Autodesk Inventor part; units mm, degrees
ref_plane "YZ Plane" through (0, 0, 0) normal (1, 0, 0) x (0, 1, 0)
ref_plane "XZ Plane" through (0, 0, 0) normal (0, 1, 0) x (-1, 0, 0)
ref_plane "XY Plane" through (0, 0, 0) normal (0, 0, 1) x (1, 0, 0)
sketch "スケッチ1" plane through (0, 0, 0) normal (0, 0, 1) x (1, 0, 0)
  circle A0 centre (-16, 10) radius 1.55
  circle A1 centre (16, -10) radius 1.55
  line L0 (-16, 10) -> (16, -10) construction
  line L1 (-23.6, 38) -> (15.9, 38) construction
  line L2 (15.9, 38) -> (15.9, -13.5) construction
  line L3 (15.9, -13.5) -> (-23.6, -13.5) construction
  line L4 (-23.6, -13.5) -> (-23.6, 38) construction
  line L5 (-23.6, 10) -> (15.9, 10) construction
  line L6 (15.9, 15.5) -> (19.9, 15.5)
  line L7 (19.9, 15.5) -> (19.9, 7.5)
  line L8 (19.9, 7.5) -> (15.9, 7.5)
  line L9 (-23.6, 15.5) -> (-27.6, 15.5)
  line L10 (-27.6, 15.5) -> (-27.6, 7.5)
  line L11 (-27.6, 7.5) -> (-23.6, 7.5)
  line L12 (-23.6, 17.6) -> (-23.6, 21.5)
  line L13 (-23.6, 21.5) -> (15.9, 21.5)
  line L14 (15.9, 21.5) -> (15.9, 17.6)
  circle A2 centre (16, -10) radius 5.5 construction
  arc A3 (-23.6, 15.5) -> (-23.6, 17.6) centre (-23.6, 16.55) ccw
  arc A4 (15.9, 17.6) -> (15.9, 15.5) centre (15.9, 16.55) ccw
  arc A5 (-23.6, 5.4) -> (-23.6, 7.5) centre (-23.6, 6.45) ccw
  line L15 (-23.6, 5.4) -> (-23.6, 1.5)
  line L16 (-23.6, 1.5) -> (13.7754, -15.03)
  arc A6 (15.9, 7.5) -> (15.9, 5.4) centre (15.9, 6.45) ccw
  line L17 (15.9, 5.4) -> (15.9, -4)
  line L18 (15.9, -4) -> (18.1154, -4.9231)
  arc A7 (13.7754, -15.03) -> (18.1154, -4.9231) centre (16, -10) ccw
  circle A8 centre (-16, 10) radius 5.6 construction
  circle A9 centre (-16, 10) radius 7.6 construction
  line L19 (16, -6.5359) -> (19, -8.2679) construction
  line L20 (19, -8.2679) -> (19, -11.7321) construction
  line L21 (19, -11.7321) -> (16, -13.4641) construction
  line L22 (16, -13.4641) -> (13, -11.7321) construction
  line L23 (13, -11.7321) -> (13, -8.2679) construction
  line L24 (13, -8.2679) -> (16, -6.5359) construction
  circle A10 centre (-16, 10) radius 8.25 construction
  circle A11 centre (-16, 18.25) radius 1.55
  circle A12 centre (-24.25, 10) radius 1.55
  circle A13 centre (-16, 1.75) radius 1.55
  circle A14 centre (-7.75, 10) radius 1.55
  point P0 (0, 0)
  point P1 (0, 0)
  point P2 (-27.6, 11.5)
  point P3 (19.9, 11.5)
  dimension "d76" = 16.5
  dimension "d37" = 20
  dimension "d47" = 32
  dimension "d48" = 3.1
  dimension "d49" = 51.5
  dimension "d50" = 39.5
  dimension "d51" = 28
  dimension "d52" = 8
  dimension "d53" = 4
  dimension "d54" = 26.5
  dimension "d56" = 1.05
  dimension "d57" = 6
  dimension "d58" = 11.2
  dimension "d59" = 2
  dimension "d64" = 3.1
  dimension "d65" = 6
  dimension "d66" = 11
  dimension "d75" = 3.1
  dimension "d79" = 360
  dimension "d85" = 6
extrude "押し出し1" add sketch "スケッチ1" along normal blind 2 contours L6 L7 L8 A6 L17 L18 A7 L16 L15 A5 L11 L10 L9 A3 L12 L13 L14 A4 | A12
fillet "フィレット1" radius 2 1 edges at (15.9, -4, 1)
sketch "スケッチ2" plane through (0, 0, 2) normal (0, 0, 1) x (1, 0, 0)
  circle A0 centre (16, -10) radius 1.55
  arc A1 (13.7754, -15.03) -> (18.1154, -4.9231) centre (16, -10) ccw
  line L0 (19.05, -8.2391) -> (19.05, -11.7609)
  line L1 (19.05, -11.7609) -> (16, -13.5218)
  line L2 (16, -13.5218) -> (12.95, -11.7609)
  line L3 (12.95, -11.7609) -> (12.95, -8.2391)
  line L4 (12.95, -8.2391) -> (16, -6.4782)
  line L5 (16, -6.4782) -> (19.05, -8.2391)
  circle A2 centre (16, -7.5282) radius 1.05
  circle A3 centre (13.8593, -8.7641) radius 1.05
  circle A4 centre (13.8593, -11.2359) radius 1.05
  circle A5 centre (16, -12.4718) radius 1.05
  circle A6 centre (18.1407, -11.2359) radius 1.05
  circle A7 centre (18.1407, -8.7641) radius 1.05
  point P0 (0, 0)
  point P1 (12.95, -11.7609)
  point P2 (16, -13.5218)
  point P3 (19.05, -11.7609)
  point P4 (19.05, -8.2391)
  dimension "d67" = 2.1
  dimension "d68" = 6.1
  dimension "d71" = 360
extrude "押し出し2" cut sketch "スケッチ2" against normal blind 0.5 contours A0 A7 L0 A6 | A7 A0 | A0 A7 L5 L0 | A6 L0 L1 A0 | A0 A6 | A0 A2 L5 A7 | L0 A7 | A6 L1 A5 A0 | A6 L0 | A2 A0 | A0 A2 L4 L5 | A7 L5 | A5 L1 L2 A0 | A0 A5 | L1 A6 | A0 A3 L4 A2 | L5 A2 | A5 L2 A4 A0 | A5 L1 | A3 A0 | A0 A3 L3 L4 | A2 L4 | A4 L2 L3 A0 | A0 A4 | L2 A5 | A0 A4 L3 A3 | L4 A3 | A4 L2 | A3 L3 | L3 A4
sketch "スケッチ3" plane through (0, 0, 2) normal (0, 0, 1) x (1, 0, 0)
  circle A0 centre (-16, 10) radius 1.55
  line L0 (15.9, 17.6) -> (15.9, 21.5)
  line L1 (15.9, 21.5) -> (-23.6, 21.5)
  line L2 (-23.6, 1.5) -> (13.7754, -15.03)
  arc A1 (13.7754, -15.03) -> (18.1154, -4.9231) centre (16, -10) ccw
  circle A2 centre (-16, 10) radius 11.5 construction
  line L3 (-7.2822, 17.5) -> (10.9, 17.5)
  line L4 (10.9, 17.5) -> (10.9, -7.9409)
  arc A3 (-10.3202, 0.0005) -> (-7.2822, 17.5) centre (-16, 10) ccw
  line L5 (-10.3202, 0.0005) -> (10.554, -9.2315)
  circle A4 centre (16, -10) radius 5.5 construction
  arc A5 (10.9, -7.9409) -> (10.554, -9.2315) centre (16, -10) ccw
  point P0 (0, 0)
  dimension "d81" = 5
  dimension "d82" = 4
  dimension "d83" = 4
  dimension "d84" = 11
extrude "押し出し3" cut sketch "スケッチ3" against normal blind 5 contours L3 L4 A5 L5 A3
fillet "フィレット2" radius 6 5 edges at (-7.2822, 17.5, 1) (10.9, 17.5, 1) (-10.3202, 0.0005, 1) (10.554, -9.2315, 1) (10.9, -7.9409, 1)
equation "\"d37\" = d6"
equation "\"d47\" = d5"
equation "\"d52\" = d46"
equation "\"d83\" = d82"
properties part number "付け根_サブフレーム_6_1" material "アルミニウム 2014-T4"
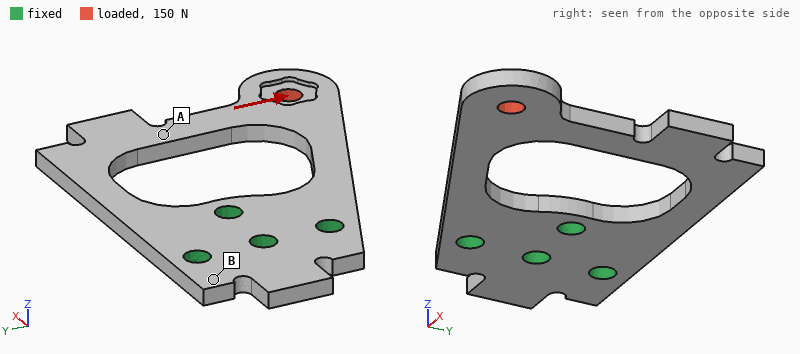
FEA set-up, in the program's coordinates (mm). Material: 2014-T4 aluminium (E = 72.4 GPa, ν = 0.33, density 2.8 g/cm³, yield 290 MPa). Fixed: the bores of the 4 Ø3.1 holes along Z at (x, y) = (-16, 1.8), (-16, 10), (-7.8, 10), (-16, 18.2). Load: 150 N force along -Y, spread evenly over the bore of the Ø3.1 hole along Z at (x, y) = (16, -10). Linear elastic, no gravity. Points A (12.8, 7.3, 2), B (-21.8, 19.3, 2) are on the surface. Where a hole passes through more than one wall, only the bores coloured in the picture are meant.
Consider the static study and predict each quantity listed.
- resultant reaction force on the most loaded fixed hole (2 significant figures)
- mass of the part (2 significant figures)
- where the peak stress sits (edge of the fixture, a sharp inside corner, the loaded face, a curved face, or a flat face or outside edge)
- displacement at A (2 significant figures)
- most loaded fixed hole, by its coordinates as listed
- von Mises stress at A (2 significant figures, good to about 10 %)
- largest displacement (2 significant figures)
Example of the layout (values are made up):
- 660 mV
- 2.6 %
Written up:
- 280 N
- 4.8 g
- a curved face
- 65 µm
- (-7.8, 10)
- 20 MPa
- 98 µm
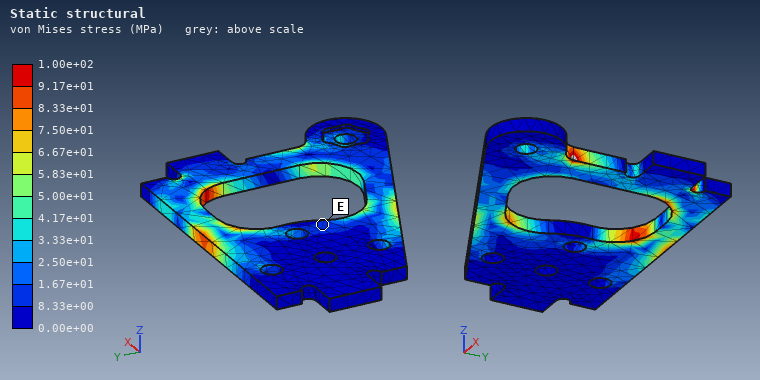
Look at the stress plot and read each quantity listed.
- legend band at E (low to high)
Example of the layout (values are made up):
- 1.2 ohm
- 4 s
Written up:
- 8.33e+00 to 1.67e+01 MPa
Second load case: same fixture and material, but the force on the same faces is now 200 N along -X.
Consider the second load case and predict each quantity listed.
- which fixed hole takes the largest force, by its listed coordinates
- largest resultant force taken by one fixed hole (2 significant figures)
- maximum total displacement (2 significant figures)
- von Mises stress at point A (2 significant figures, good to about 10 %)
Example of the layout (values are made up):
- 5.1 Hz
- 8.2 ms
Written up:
- (-16, 1.8)
- 270 N
- 84 µm
- 13 MPa
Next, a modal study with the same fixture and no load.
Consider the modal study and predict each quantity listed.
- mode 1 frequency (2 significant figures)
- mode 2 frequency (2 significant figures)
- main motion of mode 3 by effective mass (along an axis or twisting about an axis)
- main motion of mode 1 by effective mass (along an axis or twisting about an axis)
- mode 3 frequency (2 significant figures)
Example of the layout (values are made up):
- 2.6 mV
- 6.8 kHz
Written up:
- 1100 Hz
- 2400 Hz
- along Y
- along Z
- 5600 Hz
